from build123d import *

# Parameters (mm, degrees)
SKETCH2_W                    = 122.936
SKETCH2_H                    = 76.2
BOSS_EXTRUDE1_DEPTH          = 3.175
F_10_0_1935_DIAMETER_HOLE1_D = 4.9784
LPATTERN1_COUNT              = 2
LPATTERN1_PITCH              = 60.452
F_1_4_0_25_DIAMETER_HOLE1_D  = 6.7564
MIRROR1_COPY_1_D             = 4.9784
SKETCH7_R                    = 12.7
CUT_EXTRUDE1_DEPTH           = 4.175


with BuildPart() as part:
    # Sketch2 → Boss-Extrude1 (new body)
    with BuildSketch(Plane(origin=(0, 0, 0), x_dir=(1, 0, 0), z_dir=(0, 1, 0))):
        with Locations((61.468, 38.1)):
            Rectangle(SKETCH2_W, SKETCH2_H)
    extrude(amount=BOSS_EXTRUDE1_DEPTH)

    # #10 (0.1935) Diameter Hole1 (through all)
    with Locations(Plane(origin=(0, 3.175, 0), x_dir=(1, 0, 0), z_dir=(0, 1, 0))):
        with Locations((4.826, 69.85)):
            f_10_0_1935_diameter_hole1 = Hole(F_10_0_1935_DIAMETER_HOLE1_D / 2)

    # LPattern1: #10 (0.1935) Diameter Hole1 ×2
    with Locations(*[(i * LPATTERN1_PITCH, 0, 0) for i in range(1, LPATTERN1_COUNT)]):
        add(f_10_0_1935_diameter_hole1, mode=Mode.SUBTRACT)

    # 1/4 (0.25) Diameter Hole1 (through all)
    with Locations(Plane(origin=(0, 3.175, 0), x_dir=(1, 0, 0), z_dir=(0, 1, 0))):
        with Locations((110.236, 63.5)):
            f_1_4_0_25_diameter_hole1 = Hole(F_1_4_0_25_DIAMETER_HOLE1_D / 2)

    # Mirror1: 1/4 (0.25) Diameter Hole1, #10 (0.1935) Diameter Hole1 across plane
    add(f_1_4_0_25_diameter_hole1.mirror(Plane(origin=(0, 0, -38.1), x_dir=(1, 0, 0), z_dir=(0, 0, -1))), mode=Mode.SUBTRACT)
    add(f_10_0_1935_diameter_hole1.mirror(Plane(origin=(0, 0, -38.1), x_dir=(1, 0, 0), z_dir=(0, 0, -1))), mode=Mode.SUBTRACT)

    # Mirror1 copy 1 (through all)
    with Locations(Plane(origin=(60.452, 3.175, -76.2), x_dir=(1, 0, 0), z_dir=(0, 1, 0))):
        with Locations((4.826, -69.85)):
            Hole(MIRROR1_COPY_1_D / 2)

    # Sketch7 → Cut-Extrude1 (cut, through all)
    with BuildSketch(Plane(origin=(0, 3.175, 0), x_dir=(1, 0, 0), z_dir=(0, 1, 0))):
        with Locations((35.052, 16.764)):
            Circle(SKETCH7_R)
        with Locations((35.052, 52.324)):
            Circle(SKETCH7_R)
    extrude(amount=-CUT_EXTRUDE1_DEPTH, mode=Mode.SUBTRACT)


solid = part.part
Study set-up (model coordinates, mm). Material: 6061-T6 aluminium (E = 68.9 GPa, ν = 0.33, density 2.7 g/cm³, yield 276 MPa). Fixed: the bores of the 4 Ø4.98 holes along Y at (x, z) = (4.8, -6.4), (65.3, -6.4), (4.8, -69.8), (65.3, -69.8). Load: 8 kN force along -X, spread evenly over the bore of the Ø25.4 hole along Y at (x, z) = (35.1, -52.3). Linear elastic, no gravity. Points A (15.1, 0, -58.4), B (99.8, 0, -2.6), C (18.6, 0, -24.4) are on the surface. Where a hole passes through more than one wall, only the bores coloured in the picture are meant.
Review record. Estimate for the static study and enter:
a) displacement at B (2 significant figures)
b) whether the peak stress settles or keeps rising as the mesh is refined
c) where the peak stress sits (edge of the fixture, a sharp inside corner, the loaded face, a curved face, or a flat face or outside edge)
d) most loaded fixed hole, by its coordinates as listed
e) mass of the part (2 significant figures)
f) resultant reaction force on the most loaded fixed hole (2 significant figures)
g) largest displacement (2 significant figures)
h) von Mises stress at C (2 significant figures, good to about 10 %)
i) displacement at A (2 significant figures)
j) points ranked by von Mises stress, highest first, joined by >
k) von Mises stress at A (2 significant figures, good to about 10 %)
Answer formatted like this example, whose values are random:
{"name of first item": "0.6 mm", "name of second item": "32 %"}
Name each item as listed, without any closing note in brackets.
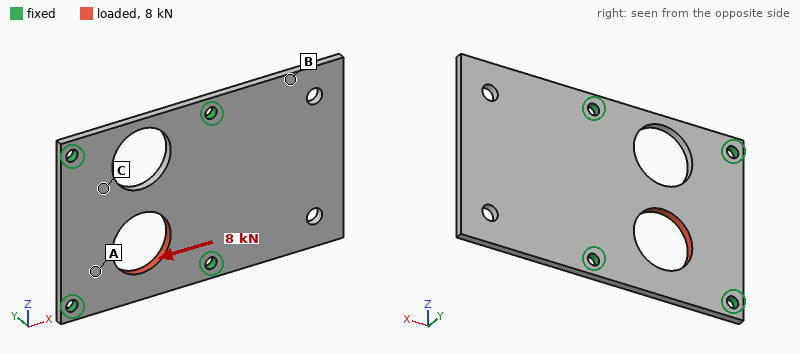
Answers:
{"displacement at B": "5.7 µm", "whether the peak stress settles or keeps rising as the mesh is refined": "keeps rising", "where the peak stress sits": "edge of the fixture", "most loaded fixed hole, by its coordinates as listed": "(65.3, -69.8)", "mass of the part": "70 g", "resultant reaction force on the most loaded fixed hole": "3.2 kN", "largest displacement": "29 µm", "von Mises stress at C": "23 MPa", "displacement at A": "18 µm", "points ranked by von Mises stress, highest first, joined by >": "A > C > B", "von Mises stress at A": "44 MPa"}
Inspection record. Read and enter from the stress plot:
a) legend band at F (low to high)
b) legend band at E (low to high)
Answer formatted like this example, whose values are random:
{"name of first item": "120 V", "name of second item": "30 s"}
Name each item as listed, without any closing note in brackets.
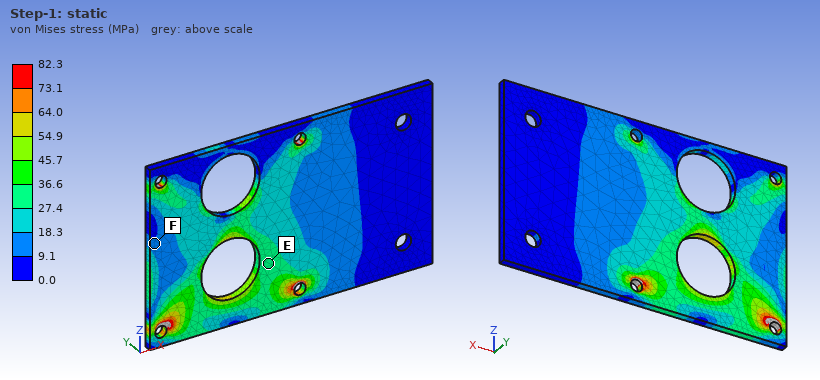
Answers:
{"legend band at F": "9.1 to 18.3 MPa", "legend band at E": "27.4 to 36.6 MPa"}
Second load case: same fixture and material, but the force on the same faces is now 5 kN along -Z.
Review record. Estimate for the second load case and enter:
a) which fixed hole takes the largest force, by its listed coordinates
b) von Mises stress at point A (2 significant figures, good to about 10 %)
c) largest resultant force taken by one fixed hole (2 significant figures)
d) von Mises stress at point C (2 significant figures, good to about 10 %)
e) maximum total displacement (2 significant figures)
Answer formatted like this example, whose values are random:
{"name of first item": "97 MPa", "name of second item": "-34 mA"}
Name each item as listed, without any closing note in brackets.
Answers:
{"which fixed hole takes the largest force, by its listed coordinates": "(65.3, -69.8)", "von Mises stress at point A": "26 MPa", "largest resultant force taken by one fixed hole": "1.6 kN", "von Mises stress at point C": "20 MPa", "maximum total displacement": "29 µm"}
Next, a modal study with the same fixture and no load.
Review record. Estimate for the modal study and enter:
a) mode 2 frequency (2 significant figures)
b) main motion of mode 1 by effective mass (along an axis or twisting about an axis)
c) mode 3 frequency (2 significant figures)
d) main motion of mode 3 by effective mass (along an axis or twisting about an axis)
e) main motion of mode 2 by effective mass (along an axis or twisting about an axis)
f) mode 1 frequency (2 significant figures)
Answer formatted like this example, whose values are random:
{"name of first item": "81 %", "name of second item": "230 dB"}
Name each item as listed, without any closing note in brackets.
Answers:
{"mode 2 frequency": "1600 Hz", "main motion of mode 1 by effective mass": "along Y", "mode 3 frequency": "3200 Hz", "main motion of mode 3 by effective mass": "along Y", "main motion of mode 2 by effective mass": "twisting about X", "mode 1 frequency": "710 Hz"}
